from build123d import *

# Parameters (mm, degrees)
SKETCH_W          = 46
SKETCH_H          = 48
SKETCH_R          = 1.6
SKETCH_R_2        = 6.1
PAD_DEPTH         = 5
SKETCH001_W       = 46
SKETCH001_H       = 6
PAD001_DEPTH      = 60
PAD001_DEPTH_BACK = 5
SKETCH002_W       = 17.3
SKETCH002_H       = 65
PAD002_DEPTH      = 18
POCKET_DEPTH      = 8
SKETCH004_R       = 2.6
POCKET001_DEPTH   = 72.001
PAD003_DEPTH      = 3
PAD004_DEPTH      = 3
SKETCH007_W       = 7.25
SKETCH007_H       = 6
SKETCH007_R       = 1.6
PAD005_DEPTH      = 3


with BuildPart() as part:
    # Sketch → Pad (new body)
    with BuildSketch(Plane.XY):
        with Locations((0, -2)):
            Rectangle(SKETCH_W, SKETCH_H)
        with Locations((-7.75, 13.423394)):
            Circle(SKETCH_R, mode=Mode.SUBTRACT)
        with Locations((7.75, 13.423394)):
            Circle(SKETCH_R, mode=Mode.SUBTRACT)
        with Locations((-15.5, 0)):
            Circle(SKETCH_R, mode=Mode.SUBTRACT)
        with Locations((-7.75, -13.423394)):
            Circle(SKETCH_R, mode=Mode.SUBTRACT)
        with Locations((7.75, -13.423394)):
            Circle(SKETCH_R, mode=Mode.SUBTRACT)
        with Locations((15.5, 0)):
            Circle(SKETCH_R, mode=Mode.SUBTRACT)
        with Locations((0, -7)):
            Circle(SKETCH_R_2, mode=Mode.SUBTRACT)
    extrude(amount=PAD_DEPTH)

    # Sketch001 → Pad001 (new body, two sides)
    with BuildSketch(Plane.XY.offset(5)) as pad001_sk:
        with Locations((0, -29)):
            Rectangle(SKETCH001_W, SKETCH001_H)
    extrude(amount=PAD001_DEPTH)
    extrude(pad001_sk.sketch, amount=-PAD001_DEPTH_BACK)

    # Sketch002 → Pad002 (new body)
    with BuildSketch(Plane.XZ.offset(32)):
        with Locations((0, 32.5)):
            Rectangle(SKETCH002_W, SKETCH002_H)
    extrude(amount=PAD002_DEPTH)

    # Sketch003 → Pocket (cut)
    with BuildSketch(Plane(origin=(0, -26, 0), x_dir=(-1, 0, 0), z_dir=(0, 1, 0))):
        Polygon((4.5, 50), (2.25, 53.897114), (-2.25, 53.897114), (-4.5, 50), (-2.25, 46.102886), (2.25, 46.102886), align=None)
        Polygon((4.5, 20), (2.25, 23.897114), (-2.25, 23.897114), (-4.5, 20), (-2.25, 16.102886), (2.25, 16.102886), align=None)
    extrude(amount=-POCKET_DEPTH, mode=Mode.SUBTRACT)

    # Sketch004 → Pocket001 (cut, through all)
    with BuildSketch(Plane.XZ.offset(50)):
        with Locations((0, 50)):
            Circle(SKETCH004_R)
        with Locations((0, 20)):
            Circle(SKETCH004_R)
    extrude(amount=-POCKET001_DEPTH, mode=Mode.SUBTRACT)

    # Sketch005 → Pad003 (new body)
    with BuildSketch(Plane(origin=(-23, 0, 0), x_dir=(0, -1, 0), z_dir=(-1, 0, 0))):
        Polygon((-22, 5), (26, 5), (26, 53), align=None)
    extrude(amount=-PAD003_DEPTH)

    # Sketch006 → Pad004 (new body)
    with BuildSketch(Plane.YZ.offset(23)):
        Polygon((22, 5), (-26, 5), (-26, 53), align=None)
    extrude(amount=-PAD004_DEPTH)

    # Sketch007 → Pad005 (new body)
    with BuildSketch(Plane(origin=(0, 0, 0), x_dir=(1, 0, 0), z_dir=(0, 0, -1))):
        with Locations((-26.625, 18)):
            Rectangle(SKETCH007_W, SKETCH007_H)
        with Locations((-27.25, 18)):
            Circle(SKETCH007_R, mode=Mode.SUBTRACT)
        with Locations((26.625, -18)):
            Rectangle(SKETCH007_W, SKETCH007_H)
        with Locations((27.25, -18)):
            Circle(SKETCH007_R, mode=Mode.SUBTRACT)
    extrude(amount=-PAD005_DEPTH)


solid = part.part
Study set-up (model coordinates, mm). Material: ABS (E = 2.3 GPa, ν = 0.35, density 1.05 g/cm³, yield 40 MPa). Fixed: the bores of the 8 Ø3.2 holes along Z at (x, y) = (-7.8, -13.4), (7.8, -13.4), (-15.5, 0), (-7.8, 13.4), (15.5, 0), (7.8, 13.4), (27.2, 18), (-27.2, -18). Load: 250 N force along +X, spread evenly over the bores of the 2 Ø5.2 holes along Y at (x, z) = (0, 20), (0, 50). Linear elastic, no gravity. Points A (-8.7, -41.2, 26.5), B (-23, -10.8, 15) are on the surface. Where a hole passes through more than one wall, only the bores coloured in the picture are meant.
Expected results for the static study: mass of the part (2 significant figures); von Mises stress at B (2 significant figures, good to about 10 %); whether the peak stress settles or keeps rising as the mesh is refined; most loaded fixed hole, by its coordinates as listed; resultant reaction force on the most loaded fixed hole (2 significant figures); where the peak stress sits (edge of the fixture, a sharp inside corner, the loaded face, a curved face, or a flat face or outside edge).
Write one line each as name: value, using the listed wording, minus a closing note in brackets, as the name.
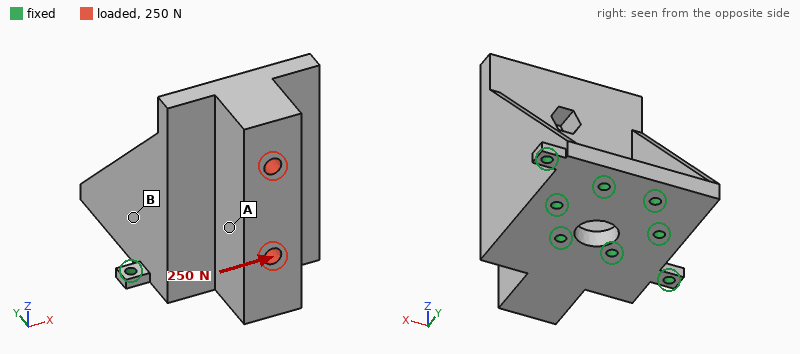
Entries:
mass of the part: 57 g
von Mises stress at B: 2.6 MPa
whether the peak stress settles or keeps rising as the mesh is refined: keeps rising
most loaded fixed hole, by its coordinates as listed: (7.8, -13.4)
resultant reaction force on the most loaded fixed hole: 190 N
where the peak stress sits: edge of the fixture
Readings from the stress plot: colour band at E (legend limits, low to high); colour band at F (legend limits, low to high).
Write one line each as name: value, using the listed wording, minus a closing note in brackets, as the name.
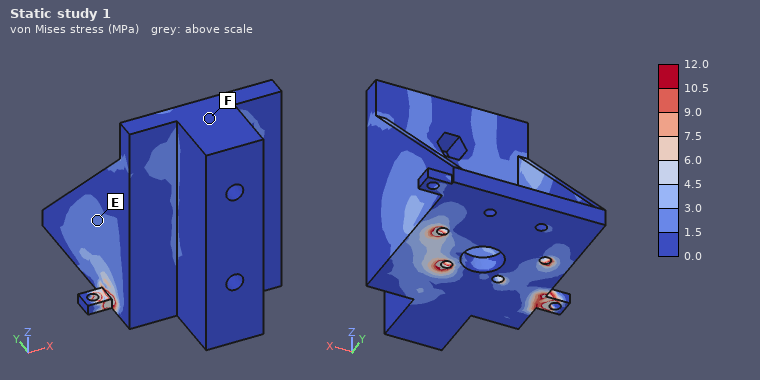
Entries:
colour band at E: 1.5 to 3.0 MPa
colour band at F: 0.0 to 1.5 MPa
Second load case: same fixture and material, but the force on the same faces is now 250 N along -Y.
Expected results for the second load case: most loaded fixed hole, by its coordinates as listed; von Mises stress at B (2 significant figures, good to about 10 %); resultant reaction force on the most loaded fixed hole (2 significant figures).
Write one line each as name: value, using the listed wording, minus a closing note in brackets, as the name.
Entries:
most loaded fixed hole, by its coordinates as listed: (-15.5, 0)
von Mises stress at B: 2.1 MPa
resultant reaction force on the most loaded fixed hole: 150 N
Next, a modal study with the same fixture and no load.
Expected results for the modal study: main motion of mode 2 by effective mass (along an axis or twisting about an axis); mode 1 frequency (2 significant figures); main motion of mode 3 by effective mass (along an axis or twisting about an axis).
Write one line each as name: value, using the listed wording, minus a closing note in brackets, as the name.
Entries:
main motion of mode 2 by effective mass: along X
mode 1 frequency: 540 Hz
main motion of mode 3 by effective mass: along Z
